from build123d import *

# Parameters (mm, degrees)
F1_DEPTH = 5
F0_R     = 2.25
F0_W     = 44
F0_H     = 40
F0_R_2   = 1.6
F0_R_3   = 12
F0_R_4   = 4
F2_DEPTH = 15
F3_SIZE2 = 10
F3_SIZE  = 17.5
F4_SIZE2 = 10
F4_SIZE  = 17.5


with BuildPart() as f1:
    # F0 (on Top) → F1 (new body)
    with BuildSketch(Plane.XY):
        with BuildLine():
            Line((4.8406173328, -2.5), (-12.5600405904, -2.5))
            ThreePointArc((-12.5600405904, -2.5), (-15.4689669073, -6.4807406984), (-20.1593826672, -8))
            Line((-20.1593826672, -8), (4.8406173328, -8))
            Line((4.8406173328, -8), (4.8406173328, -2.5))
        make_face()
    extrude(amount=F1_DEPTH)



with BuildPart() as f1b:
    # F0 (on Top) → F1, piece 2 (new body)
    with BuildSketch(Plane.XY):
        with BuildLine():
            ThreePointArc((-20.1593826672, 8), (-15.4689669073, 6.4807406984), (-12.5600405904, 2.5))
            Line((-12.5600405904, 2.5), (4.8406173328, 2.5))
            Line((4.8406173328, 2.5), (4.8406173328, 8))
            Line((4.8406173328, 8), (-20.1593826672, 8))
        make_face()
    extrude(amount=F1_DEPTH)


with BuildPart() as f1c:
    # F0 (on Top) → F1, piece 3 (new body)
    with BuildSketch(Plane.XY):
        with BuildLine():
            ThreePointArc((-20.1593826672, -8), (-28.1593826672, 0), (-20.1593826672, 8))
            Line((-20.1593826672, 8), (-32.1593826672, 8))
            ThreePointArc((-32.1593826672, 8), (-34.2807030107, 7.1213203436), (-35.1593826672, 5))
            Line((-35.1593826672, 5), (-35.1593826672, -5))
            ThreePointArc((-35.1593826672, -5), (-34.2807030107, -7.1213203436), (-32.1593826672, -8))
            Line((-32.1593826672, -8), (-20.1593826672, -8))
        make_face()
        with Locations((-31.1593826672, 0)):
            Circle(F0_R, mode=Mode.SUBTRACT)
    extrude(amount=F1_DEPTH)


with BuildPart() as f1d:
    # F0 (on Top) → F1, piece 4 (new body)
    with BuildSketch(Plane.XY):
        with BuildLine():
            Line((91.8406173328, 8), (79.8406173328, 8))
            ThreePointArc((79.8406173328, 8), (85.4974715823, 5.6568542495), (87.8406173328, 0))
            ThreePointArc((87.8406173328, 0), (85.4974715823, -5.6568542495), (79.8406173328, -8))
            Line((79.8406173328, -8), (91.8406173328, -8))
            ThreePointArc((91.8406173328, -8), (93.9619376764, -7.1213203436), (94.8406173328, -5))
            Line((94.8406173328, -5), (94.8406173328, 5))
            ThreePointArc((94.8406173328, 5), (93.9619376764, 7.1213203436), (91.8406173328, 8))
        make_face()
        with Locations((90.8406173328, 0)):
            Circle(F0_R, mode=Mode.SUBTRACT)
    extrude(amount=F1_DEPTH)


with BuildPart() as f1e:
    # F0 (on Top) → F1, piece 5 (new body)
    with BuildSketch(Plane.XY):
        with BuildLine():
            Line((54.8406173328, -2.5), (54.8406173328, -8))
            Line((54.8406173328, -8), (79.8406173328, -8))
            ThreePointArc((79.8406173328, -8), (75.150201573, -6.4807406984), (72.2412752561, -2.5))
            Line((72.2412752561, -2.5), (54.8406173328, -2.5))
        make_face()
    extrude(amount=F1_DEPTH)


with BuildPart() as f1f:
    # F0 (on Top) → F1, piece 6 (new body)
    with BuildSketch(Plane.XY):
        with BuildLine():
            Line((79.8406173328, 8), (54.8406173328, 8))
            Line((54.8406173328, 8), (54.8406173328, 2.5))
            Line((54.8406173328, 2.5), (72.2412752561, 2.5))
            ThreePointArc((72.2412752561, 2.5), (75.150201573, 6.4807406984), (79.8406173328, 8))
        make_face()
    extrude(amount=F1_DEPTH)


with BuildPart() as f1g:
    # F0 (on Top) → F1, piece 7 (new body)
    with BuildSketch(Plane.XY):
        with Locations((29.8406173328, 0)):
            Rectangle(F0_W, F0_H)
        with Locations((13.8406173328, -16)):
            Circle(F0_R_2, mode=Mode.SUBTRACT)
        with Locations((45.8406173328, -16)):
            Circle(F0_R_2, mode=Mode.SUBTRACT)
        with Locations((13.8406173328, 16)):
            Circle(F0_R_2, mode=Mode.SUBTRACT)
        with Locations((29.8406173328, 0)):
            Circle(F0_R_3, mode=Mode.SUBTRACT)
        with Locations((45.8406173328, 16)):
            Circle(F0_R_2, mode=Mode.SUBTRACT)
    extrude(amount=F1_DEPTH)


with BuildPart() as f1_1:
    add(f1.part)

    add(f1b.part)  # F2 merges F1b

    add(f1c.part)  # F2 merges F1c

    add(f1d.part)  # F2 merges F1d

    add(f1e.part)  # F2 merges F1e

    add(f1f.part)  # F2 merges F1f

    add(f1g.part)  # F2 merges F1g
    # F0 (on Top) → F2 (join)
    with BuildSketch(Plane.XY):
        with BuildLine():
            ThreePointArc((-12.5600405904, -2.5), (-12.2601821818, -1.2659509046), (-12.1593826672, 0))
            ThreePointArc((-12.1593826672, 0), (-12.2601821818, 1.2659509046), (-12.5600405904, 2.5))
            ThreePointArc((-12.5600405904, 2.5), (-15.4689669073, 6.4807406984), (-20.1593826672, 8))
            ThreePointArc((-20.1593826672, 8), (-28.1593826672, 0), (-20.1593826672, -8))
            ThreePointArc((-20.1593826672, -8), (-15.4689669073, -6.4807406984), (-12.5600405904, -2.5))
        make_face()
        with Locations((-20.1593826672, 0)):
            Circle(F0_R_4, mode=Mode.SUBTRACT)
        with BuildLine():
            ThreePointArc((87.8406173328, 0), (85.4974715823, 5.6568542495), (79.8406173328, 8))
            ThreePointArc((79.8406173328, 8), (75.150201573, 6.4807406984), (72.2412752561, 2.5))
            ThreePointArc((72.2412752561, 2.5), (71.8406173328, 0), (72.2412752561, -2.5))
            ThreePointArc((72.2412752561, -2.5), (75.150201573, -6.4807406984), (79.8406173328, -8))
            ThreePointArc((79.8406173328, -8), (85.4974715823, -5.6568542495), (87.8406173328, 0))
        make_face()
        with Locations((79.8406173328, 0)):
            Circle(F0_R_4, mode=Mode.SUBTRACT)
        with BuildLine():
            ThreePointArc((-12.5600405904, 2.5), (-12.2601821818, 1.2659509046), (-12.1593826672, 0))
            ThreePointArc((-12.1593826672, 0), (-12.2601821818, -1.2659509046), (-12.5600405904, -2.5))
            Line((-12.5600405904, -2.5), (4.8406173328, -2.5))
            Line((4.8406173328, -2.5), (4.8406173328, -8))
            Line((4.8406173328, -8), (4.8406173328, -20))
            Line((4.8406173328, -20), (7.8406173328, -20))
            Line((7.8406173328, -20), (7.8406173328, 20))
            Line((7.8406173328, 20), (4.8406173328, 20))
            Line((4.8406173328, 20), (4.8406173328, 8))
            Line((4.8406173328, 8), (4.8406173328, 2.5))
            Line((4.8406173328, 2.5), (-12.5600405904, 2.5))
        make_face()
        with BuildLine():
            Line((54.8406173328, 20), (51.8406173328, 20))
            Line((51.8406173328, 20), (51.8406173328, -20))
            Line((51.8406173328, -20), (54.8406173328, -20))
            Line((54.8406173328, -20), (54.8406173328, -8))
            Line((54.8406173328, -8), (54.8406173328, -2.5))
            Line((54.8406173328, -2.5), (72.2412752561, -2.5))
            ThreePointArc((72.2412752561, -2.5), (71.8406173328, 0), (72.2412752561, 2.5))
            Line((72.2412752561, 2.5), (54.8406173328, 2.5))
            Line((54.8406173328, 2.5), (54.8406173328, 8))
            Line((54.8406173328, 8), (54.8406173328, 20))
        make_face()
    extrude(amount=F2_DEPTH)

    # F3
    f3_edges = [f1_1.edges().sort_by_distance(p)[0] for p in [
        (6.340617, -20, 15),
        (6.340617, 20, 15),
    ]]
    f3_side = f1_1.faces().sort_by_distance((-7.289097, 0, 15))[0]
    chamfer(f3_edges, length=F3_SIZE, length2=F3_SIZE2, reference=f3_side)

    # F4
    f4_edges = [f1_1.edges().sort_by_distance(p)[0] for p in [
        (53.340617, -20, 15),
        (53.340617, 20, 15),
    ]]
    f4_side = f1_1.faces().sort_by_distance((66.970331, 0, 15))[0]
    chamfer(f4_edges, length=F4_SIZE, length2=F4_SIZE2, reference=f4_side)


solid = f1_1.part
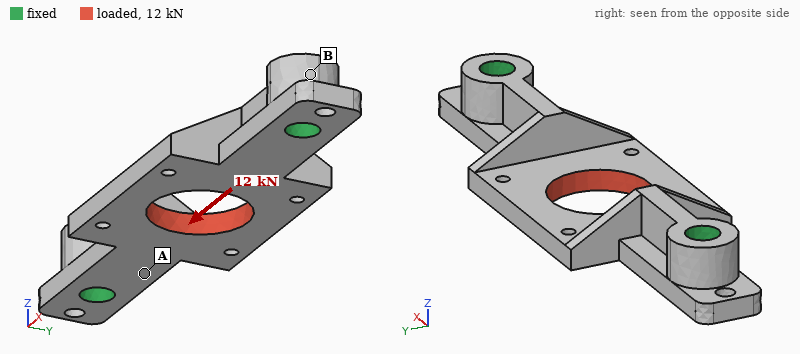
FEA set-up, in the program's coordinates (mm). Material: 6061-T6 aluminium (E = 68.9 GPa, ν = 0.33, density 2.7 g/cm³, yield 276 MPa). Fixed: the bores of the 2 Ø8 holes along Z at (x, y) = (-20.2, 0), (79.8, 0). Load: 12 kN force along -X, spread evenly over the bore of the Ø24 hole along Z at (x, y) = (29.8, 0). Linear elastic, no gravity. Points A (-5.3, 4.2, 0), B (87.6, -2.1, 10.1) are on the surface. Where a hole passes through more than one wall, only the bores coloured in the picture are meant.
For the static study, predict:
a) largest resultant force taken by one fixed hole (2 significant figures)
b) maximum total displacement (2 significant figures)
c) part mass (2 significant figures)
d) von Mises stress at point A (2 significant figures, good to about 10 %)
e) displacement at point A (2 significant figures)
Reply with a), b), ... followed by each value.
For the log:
a) 6.0 kN
b) 46 µm
c) 52 g
d) 69 MPa
e) 14 µm
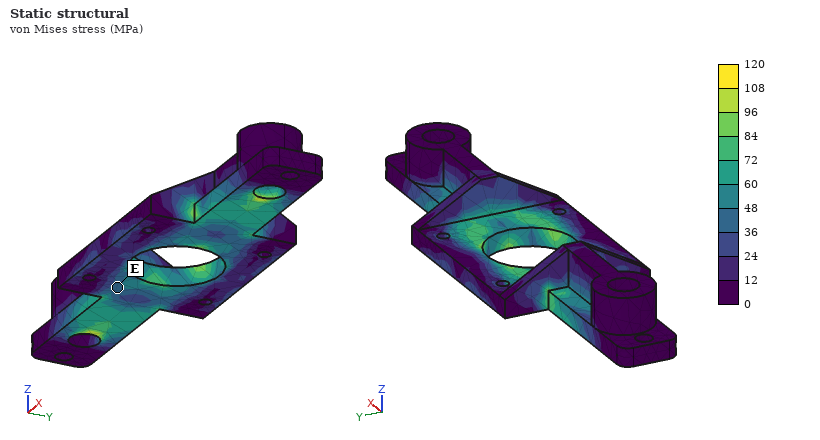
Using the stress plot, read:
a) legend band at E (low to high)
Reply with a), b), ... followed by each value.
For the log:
a) 36 to 48 MPa
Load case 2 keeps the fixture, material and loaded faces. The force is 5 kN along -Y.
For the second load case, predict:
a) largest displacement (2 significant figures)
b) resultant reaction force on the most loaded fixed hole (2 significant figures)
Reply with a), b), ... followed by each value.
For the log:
a) 0.11 mm
b) 2.5 kN
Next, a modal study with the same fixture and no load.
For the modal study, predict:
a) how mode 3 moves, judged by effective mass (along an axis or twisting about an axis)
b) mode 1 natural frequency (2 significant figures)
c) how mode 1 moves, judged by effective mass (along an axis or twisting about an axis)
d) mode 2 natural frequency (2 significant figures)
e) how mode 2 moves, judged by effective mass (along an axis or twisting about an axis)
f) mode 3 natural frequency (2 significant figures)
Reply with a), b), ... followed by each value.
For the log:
a) along Y
b) 4400 Hz
c) twisting about X
d) 5200 Hz
e) along Z
f) 8000 Hz
